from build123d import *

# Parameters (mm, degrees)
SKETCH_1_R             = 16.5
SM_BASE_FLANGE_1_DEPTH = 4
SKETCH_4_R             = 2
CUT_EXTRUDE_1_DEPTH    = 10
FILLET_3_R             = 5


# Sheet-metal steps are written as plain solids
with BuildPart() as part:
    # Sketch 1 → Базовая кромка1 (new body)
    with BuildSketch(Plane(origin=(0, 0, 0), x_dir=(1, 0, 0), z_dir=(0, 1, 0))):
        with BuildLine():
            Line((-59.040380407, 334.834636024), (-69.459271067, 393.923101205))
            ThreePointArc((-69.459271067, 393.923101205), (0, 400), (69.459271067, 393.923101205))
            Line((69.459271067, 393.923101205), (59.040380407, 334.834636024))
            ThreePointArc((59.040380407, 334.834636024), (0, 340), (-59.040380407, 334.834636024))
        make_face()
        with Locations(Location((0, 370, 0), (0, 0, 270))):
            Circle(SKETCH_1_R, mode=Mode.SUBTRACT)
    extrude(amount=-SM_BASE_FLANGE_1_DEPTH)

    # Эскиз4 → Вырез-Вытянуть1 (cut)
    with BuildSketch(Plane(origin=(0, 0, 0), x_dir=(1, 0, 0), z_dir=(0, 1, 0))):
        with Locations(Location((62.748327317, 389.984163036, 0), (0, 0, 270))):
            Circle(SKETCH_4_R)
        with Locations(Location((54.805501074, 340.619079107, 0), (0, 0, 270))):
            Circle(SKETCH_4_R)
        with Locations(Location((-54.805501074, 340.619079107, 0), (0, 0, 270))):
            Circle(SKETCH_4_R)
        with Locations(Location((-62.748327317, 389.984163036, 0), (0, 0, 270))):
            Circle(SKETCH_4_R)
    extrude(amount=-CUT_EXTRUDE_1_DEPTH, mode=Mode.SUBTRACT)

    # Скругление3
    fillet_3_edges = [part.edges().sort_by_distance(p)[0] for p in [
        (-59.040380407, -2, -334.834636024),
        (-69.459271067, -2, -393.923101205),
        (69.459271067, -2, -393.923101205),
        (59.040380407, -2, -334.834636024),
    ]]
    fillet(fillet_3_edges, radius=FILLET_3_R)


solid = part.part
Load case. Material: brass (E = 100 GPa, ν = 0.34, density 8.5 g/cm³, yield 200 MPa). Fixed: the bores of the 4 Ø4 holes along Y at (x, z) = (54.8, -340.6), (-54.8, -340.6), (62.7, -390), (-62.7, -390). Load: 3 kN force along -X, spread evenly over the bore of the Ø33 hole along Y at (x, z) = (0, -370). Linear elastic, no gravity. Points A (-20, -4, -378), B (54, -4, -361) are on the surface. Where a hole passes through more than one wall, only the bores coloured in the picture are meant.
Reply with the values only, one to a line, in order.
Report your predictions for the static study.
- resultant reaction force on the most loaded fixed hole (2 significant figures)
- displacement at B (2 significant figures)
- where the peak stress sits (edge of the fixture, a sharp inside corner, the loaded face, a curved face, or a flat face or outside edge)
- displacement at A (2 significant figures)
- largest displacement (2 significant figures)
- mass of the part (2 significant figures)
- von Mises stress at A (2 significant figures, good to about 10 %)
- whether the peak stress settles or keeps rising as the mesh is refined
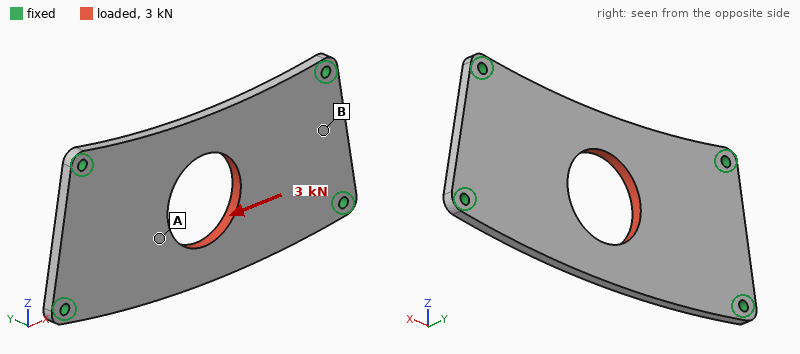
860 N
2.8 µm
edge of the fixture
4.4 µm
5.7 µm
230 g
7.9 MPa
keeps rising
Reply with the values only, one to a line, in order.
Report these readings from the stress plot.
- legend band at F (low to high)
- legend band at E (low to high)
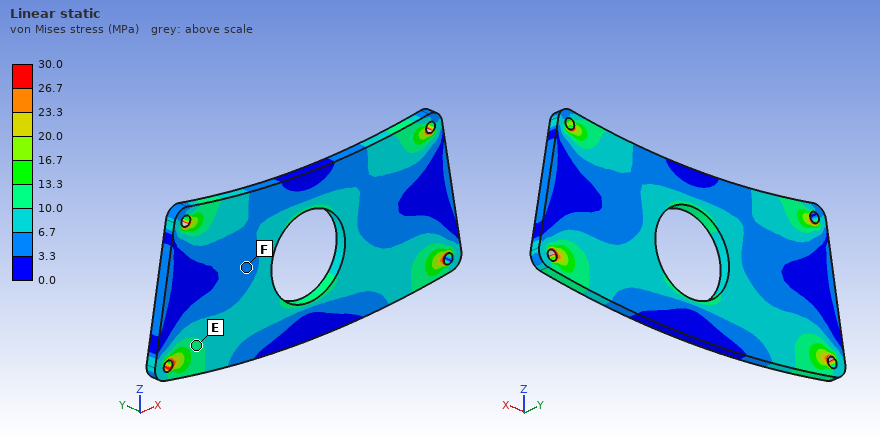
3.3 to 6.7 MPa
10.0 to 13.3 MPa
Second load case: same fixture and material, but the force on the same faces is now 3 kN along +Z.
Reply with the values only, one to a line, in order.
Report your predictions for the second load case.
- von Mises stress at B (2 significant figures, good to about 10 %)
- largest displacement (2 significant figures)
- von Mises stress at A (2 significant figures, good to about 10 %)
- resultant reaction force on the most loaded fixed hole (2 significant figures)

8.0 MPa
15 µm
15 MPa
1.3 kN
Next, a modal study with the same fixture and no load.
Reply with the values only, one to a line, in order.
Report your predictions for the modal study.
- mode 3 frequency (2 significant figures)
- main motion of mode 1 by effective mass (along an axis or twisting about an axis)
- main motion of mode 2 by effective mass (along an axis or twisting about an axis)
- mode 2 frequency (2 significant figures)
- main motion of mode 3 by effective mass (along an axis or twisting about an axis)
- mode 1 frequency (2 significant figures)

2300 Hz
along Y
twisting about X
1700 Hz
twisting about Z
900 Hz
